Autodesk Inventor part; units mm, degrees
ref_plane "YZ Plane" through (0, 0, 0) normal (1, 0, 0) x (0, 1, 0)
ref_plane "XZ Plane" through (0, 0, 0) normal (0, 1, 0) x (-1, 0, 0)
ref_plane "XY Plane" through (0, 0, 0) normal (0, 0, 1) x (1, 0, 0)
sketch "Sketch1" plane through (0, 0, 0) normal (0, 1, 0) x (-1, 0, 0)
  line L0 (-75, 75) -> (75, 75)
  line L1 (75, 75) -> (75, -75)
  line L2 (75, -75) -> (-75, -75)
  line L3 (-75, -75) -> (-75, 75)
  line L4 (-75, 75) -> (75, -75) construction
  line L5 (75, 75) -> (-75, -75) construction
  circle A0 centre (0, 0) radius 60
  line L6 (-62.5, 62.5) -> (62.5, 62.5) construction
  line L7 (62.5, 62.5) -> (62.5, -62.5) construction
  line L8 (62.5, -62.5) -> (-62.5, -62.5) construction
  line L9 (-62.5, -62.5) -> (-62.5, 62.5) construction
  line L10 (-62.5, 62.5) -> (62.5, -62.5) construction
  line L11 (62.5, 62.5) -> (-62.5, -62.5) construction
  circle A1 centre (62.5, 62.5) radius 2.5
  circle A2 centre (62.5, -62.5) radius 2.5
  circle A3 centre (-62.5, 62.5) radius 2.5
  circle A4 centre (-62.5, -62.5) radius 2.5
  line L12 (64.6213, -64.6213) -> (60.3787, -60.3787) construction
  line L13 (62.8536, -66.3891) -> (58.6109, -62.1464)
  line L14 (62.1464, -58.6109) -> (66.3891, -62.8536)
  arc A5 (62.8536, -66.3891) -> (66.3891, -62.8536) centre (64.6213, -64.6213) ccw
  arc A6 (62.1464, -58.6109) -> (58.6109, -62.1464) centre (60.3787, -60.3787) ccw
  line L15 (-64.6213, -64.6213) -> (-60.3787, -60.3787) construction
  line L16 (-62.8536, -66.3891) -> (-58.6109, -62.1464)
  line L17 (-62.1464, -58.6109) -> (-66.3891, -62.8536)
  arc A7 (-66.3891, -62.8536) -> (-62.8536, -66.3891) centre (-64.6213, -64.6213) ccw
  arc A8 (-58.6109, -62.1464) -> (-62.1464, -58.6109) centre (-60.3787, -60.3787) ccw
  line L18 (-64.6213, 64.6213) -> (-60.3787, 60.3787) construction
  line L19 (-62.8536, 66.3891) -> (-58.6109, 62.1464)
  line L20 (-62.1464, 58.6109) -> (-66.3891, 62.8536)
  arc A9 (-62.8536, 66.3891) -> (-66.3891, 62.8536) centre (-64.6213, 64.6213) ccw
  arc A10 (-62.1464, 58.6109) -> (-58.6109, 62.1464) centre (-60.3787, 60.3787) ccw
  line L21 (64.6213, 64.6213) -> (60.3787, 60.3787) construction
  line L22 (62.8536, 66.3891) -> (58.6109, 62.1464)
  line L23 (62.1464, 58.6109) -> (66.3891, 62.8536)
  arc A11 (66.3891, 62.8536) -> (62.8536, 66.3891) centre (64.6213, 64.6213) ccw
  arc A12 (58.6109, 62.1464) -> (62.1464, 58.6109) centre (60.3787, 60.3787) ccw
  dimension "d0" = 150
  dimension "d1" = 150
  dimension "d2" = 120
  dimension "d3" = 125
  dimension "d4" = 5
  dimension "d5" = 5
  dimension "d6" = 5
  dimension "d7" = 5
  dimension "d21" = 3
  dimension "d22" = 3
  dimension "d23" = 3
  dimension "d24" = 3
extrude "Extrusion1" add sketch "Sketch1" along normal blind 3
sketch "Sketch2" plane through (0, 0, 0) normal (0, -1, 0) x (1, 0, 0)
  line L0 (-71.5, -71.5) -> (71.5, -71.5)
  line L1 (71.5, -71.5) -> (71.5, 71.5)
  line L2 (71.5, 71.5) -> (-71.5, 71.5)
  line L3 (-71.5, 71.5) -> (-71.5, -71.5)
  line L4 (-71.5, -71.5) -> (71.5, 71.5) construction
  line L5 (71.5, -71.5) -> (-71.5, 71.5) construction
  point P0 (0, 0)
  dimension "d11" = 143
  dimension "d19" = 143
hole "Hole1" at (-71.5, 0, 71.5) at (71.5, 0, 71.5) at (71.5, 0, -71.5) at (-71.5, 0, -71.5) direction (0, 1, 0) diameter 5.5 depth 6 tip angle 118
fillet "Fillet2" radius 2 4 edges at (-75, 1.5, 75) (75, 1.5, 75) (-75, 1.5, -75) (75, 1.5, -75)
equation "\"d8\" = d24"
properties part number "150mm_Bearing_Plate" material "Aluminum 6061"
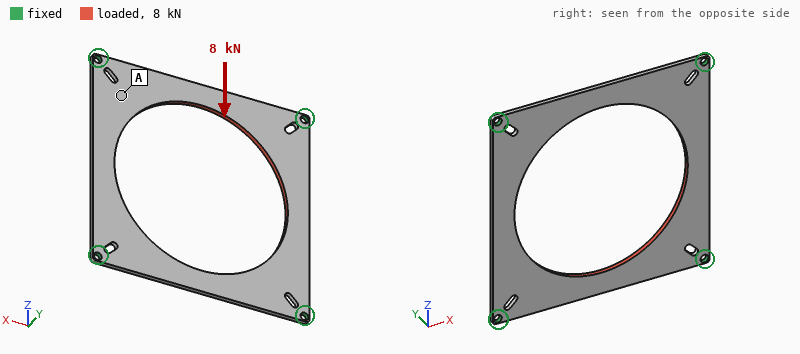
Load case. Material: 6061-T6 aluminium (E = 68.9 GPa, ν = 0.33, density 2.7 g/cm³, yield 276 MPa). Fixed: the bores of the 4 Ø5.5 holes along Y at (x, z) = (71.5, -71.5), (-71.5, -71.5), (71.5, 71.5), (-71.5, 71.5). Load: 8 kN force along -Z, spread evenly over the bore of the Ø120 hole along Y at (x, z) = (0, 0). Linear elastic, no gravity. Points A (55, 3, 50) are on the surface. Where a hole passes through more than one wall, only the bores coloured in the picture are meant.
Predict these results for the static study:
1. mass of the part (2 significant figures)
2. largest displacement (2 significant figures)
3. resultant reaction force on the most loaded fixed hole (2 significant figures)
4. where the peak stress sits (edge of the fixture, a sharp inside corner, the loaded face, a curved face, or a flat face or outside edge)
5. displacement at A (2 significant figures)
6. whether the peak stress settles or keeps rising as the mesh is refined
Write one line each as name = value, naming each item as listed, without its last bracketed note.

mass of the part = 88 g
largest displacement = 0.15 mm
resultant reaction force on the most loaded fixed hole = 2.1 kN
where the peak stress sits = edge of the fixture
displacement at A = 0.054 mm
whether the peak stress settles or keeps rising as the mesh is refined = keeps rising
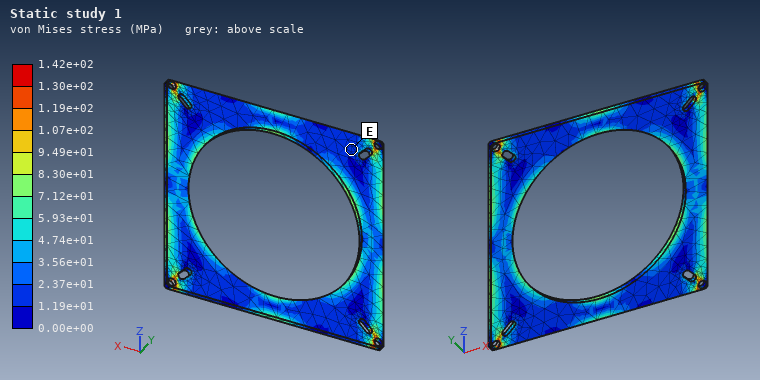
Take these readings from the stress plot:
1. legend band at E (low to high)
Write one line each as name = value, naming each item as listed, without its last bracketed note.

legend band at E = 1.19e+01 to 2.37e+01 MPa
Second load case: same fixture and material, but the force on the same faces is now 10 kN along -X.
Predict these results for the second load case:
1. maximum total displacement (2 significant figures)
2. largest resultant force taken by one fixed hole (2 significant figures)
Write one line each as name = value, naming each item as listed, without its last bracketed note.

maximum total displacement = 0.19 mm
largest resultant force taken by one fixed hole = 2.7 kN
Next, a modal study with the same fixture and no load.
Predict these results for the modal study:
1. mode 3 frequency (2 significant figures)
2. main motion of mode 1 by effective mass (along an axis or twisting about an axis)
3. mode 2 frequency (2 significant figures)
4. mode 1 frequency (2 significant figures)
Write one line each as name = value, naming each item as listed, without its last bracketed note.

mode 3 frequency = 800 Hz
main motion of mode 1 by effective mass = along Y
mode 2 frequency = 800 Hz
mode 1 frequency = 670 Hz
